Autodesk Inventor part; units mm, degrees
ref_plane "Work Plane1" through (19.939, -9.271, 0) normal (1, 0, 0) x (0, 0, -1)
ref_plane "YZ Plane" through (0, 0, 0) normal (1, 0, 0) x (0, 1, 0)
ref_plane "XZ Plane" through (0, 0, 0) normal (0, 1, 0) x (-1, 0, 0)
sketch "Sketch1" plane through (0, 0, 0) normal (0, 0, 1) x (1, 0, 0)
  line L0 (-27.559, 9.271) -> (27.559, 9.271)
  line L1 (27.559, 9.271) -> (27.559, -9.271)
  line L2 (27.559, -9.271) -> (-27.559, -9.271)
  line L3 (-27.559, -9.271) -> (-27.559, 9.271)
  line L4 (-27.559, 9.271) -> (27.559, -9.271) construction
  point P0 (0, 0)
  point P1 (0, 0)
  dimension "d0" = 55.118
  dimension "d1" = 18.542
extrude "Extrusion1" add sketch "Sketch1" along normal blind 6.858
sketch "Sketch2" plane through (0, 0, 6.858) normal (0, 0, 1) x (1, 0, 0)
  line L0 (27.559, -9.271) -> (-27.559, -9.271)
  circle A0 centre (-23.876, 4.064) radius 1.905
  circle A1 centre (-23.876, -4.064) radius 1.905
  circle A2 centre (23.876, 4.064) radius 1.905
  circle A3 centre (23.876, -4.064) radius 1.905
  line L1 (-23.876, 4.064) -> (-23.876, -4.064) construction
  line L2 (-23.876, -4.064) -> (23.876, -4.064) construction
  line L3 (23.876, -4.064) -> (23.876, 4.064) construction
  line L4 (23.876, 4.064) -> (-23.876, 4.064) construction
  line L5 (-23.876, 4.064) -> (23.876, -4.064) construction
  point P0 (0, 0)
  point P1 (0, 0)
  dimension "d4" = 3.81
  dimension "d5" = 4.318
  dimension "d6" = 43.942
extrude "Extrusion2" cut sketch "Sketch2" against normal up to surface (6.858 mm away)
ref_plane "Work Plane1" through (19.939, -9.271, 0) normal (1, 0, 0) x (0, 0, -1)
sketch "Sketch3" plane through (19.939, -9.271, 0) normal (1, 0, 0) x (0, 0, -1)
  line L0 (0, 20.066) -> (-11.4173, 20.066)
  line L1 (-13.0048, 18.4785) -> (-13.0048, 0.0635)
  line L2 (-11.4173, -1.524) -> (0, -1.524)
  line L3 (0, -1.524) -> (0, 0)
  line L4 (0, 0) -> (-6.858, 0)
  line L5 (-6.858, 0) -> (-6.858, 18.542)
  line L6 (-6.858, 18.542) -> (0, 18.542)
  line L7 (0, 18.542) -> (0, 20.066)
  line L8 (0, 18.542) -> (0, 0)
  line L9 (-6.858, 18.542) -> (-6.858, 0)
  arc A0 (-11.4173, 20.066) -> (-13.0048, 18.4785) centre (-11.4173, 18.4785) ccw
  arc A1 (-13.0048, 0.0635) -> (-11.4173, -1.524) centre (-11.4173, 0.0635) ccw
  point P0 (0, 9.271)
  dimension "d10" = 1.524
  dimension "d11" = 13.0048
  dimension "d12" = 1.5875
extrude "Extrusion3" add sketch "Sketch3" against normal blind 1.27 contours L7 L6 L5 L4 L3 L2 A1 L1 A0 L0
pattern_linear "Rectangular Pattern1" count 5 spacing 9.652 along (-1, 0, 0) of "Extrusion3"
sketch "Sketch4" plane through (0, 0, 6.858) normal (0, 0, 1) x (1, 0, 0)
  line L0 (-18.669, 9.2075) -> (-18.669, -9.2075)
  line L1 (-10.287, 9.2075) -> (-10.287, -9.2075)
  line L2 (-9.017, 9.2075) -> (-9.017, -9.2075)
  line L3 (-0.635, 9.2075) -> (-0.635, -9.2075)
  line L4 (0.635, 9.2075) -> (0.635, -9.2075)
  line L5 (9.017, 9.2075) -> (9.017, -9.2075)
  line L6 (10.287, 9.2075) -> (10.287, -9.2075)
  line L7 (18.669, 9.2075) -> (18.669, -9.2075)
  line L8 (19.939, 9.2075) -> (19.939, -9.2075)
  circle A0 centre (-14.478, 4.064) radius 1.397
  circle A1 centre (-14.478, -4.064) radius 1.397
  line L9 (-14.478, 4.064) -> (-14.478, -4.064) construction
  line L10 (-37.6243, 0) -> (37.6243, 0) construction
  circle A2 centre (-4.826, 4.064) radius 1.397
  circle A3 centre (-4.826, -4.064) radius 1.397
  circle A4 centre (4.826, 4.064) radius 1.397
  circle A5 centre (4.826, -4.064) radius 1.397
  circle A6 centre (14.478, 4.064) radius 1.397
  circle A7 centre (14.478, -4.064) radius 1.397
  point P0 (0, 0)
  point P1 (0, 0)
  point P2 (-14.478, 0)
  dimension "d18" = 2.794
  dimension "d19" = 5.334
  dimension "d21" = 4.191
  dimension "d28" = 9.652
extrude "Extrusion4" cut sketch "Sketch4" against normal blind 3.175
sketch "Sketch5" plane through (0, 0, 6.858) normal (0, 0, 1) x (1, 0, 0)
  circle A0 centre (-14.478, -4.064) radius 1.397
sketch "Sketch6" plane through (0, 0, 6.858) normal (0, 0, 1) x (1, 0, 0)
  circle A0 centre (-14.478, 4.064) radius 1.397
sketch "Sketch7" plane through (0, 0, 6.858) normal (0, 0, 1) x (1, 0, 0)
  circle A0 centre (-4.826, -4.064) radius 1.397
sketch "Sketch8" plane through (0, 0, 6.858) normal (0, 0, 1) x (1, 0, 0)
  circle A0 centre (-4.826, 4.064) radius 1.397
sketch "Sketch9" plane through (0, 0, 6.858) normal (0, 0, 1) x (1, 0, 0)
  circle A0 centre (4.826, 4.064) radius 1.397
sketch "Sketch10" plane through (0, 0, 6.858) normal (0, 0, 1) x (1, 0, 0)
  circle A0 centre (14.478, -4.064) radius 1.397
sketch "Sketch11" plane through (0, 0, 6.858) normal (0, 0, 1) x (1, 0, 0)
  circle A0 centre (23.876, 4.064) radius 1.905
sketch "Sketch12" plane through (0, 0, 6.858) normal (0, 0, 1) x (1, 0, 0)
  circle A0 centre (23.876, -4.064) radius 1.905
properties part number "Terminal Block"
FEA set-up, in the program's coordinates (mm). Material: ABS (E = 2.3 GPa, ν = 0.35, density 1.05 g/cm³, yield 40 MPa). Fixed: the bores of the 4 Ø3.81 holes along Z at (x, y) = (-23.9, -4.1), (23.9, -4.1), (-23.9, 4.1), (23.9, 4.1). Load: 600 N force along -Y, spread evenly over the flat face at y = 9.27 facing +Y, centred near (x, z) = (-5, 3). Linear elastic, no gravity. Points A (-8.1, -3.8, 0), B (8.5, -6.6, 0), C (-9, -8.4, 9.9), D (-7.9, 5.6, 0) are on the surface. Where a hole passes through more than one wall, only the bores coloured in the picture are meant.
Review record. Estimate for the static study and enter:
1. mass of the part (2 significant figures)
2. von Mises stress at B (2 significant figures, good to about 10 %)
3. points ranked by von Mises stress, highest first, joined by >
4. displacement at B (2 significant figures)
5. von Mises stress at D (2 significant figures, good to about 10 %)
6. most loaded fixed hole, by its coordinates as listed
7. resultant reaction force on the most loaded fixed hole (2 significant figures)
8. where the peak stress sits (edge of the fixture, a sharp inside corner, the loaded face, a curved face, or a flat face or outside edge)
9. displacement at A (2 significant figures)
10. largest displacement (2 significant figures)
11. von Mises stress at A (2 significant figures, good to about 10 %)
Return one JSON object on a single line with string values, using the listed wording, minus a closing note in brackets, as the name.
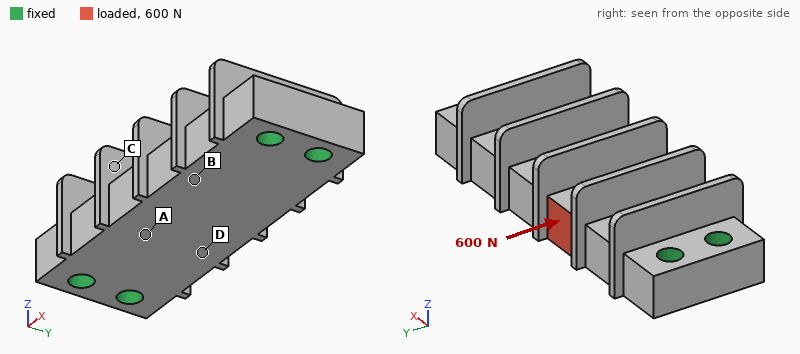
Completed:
{"mass of the part": "7.9 g", "von Mises stress at B": "2.7 MPa", "points ranked by von Mises stress, highest first, joined by >": "D > A > B > C", "displacement at B": "0.067 mm", "von Mises stress at D": "8.6 MPa", "most loaded fixed hole, by its coordinates as listed": "(-23.9, -4.1)", "resultant reaction force on the most loaded fixed hole": "350 N", "where the peak stress sits": "a curved face", "displacement at A": "0.088 mm", "largest displacement": "0.14 mm", "von Mises stress at A": "4.8 MPa"}
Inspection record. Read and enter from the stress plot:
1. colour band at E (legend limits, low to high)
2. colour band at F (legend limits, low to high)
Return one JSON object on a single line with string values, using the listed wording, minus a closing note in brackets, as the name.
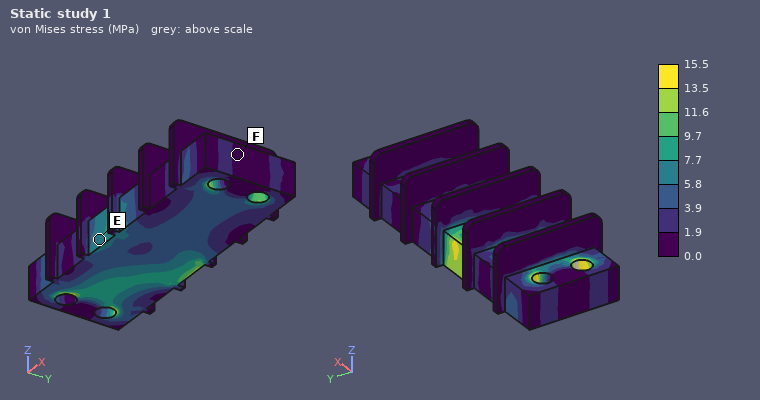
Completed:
{"colour band at E": "5.8 to 7.7 MPa", "colour band at F": "0.0 to 1.9 MPa"}
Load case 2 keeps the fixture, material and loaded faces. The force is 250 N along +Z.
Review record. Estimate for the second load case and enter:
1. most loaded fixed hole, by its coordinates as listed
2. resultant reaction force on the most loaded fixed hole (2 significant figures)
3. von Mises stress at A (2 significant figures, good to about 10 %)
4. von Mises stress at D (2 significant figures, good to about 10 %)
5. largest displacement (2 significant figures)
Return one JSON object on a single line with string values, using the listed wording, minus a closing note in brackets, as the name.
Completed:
{"most loaded fixed hole, by its coordinates as listed": "(-23.9, 4.1)", "resultant reaction force on the most loaded fixed hole": "170 N", "von Mises stress at A": "5.3 MPa", "von Mises stress at D": "14 MPa", "largest displacement": "0.31 mm"}
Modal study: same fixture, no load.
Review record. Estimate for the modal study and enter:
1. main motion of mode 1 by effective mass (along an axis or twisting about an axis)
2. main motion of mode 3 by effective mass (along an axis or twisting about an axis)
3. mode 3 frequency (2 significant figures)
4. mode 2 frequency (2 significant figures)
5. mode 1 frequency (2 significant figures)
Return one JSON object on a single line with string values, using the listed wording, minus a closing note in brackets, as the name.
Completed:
{"main motion of mode 1 by effective mass": "along Z", "main motion of mode 3 by effective mass": "along Y", "mode 3 frequency": "6600 Hz", "mode 2 frequency": "5400 Hz", "mode 1 frequency": "4000 Hz"}
